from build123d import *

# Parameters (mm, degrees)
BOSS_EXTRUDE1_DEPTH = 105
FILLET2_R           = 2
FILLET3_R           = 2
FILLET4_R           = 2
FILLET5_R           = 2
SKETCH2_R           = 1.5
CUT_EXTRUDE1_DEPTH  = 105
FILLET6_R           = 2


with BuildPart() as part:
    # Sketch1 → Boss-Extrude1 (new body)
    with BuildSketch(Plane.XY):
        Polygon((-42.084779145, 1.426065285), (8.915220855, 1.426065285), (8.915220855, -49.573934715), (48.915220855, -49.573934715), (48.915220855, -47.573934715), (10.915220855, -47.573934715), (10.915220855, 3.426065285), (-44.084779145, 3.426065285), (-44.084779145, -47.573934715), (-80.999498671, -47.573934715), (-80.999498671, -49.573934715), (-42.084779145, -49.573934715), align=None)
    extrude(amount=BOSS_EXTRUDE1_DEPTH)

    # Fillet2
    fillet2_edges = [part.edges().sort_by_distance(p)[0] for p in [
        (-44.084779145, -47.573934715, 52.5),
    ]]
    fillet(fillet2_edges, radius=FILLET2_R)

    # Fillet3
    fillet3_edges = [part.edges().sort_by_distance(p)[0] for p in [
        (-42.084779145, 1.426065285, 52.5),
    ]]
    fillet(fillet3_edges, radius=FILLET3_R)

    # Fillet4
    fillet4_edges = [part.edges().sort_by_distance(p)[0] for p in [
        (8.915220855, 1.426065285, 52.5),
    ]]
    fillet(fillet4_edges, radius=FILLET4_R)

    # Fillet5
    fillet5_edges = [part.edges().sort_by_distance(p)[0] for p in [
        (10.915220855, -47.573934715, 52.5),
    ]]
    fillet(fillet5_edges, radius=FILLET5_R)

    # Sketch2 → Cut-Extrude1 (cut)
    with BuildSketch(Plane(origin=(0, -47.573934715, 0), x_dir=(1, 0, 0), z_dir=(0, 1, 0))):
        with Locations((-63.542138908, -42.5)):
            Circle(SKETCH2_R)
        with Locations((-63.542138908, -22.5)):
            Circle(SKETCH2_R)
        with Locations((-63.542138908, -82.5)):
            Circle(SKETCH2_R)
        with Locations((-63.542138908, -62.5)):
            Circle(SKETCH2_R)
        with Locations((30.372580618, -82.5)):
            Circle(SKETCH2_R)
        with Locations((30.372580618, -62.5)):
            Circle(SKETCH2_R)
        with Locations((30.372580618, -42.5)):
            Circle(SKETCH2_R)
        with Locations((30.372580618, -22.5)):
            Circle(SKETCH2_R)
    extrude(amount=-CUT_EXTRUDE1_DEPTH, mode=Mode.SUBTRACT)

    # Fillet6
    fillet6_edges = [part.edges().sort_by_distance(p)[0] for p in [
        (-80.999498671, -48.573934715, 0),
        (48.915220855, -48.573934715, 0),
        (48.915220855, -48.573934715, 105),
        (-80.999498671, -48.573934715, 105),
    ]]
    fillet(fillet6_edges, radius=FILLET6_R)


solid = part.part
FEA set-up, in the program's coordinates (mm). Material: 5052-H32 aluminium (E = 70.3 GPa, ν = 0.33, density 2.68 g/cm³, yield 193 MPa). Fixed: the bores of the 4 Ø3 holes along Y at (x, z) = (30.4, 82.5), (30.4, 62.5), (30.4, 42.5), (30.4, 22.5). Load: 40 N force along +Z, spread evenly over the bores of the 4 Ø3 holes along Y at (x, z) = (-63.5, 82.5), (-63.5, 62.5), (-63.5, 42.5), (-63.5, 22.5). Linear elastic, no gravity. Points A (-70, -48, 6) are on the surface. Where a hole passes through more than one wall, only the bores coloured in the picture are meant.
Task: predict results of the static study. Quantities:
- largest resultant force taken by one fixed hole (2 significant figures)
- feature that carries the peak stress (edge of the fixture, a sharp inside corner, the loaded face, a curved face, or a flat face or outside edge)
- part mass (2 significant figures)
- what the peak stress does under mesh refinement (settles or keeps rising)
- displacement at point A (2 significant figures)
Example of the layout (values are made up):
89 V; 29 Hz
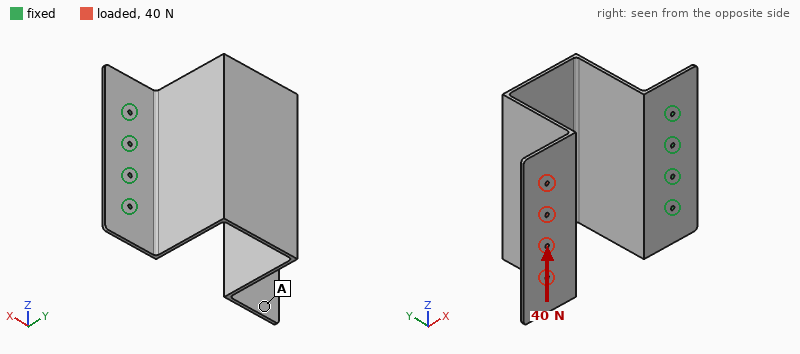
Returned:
60 N; edge of the fixture; 130 g; keeps rising; 1.7 mm
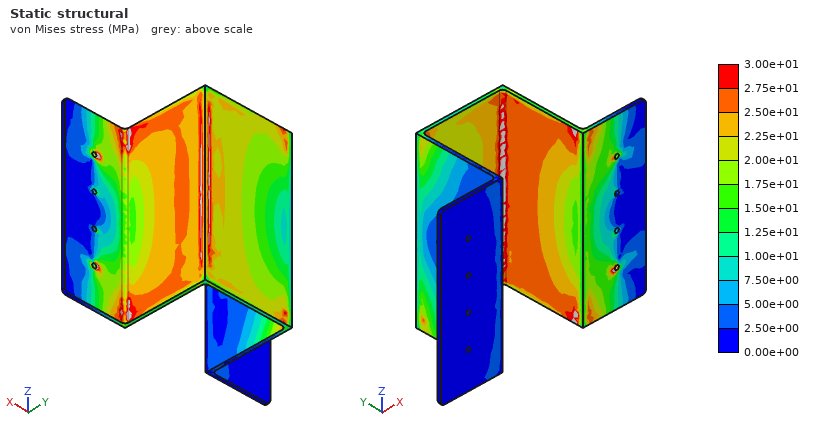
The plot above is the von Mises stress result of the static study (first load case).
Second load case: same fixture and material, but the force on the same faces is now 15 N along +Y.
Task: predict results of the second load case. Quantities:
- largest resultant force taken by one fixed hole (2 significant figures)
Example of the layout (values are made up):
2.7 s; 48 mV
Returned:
6.9 N
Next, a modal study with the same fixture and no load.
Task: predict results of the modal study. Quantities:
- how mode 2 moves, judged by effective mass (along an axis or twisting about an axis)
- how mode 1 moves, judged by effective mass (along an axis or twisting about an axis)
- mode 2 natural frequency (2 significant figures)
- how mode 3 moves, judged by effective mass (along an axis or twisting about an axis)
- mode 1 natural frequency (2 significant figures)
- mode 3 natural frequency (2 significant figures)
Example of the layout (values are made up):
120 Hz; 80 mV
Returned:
along Z; along Y; 130 Hz; along X; 71 Hz; 150 Hz
